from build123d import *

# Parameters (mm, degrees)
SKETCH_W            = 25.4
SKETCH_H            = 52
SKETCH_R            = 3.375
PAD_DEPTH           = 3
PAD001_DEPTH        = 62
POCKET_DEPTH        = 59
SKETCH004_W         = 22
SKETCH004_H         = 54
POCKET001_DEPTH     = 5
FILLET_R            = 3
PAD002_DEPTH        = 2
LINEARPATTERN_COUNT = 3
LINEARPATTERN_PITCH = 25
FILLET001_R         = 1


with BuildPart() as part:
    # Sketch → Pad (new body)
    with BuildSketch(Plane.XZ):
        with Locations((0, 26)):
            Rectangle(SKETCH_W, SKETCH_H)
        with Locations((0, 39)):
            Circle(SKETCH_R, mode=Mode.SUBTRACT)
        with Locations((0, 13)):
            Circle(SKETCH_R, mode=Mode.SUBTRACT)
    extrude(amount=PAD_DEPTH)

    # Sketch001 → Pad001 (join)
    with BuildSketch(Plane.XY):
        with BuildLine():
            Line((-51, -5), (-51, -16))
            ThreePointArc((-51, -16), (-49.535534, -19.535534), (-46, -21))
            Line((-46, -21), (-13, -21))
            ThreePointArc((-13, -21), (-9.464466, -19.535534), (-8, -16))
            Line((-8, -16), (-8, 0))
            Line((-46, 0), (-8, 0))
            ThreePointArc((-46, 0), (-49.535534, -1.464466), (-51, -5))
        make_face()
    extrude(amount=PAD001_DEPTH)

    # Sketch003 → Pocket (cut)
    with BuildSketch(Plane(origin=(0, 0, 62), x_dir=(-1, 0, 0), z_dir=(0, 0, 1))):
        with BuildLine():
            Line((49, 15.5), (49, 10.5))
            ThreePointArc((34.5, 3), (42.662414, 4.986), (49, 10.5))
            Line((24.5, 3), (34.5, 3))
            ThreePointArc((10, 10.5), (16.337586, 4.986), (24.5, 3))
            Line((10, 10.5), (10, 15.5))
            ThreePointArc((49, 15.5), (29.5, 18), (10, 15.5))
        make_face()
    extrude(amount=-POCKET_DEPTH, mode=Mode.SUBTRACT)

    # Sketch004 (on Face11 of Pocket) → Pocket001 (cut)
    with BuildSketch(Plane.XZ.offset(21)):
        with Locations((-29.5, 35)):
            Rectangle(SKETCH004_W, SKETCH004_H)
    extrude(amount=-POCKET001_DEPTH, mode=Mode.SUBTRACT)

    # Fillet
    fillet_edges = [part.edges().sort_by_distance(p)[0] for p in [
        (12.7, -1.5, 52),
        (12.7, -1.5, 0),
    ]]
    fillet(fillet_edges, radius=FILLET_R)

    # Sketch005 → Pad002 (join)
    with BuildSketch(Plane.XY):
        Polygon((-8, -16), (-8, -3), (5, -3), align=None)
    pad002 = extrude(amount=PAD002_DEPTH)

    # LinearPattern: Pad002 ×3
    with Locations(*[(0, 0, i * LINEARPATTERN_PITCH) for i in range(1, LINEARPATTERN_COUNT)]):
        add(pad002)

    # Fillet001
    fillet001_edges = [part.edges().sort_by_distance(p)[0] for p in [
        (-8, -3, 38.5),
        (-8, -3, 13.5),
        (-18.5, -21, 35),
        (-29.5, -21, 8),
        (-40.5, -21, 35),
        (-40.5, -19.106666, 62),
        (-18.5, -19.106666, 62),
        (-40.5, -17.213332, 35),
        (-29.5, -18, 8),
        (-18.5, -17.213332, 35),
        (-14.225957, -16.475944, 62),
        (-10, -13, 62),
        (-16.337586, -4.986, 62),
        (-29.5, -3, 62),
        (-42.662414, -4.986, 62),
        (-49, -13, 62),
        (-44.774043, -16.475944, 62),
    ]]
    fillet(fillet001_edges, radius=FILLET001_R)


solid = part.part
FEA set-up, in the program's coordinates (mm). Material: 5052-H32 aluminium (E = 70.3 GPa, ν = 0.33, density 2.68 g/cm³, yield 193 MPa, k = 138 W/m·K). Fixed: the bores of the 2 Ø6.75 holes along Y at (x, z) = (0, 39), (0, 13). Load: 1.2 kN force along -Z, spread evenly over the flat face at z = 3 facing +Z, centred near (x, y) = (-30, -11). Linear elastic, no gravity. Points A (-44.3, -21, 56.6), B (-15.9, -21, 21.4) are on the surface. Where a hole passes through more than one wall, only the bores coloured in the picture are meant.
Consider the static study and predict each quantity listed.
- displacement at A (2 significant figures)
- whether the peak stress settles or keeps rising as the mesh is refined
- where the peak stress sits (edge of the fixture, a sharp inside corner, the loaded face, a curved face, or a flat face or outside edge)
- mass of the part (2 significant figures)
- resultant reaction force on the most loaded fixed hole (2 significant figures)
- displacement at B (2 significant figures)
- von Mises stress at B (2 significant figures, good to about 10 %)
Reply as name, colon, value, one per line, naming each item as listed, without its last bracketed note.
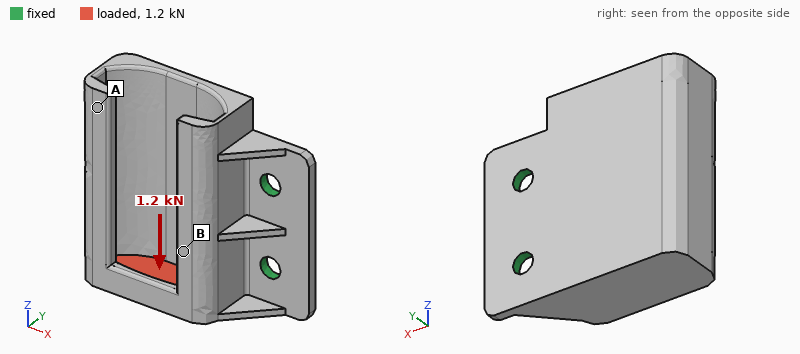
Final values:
displacement at A: 81 µm
whether the peak stress settles or keeps rising as the mesh is refined: keeps rising
where the peak stress sits: a sharp inside corner
mass of the part: 69 g
resultant reaction force on the most loaded fixed hole: 1.3 kN
displacement at B: 21 µm
von Mises stress at B: 11 MPa
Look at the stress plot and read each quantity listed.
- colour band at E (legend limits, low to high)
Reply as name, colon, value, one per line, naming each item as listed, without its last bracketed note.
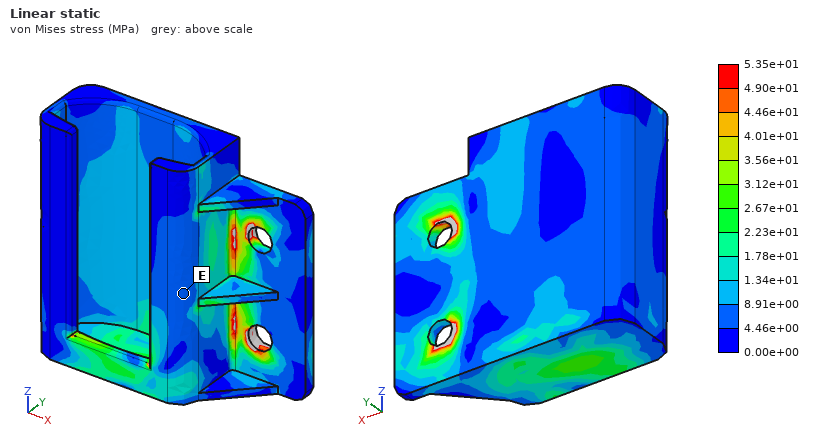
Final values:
colour band at E: 4.46e+00 to 8.91e+00 MPa
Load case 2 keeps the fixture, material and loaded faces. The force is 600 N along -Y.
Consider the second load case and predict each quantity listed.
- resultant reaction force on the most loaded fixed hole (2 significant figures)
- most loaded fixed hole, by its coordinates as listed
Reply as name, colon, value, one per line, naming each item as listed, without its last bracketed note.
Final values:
resultant reaction force on the most loaded fixed hole: 770 N
most loaded fixed hole, by its coordinates as listed: (0, 13)
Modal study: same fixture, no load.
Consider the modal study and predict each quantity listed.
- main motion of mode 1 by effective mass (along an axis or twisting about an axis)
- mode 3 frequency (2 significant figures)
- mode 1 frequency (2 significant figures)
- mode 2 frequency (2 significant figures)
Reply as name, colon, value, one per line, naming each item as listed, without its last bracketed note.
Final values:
main motion of mode 1 by effective mass: along Y
mode 3 frequency: 4300 Hz
mode 1 frequency: 960 Hz
mode 2 frequency: 2400 Hz
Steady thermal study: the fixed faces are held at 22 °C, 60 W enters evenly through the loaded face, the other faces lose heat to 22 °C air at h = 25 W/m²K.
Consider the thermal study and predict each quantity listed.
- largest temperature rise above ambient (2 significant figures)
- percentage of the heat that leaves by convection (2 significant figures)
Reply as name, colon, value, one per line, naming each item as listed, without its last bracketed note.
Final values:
largest temperature rise above ambient: 70 K
percentage of the heat that leaves by convection: 19 %
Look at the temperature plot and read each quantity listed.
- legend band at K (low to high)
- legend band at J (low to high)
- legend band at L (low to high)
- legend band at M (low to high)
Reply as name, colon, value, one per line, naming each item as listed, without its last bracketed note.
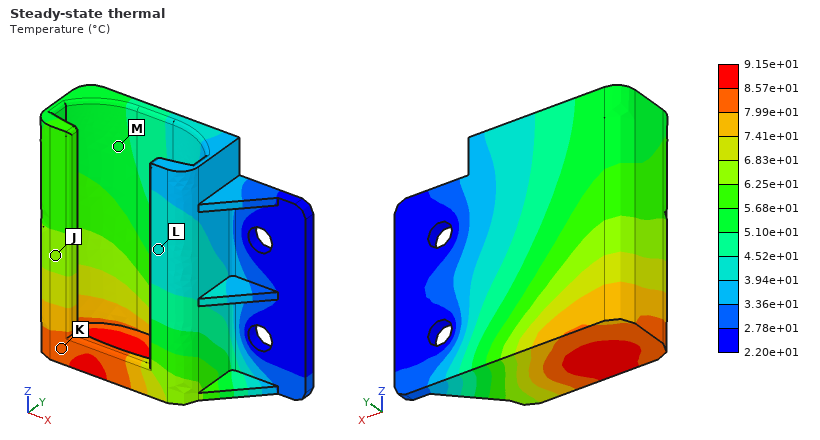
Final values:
legend band at K: 7.99e+01 to 8.57e+01 °C
legend band at J: 6.25e+01 to 6.83e+01 °C
legend band at L: 3.94e+01 to 4.52e+01 °C
legend band at M: 5.10e+01 to 5.68e+01 °C
